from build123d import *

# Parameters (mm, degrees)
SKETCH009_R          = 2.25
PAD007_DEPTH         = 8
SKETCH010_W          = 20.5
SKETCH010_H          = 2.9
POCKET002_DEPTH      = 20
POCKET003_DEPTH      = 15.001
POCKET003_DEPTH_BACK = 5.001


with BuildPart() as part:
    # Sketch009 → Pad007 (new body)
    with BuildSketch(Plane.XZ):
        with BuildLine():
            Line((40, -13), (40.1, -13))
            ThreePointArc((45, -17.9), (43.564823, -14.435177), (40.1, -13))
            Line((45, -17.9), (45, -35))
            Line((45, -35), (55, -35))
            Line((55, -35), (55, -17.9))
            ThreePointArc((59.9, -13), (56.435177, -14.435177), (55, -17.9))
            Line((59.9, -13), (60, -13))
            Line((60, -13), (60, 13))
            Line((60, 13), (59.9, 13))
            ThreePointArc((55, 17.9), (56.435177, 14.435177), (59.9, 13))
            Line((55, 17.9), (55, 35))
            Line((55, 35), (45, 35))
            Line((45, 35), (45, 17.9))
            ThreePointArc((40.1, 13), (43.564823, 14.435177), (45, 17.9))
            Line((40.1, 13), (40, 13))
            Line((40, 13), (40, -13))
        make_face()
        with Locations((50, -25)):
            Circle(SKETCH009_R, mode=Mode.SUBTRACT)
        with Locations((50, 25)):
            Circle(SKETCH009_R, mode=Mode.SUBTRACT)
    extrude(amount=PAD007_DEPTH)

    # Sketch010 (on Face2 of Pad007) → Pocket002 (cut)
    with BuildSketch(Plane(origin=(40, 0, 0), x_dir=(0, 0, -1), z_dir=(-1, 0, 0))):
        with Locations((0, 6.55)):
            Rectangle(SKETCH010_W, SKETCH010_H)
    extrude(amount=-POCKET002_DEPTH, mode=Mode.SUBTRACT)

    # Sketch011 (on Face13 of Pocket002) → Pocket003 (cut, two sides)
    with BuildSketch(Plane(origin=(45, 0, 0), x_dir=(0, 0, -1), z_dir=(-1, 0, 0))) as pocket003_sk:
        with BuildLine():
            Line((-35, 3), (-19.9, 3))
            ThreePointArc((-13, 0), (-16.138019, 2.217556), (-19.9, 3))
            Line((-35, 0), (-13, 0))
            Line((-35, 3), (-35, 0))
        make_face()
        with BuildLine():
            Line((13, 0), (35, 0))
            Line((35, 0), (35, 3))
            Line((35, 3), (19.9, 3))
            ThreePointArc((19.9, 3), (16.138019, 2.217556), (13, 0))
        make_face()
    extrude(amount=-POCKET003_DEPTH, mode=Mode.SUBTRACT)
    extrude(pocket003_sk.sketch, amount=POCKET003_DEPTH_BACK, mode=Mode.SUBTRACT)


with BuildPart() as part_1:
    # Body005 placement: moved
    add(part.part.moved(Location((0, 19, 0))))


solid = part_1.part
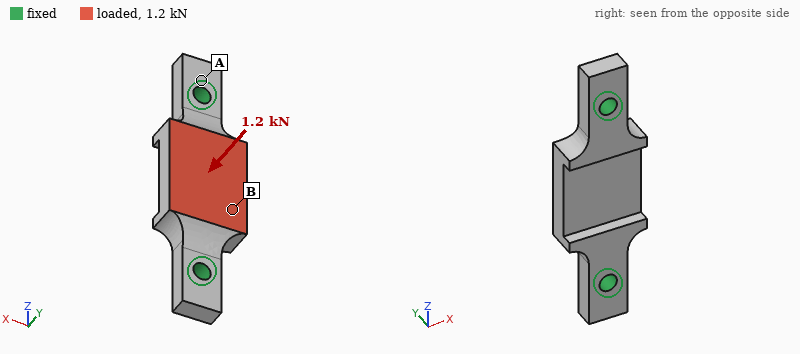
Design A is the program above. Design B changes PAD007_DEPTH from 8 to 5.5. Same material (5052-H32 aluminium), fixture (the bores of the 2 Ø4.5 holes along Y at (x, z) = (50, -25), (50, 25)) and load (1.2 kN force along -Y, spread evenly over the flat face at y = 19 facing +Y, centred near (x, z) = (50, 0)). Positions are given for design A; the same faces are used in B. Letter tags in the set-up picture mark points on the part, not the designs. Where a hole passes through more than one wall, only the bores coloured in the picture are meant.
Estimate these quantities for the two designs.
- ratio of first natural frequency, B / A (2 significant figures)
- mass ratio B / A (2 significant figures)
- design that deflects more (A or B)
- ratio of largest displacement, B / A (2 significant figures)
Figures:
0.57
0.75
B
2.5
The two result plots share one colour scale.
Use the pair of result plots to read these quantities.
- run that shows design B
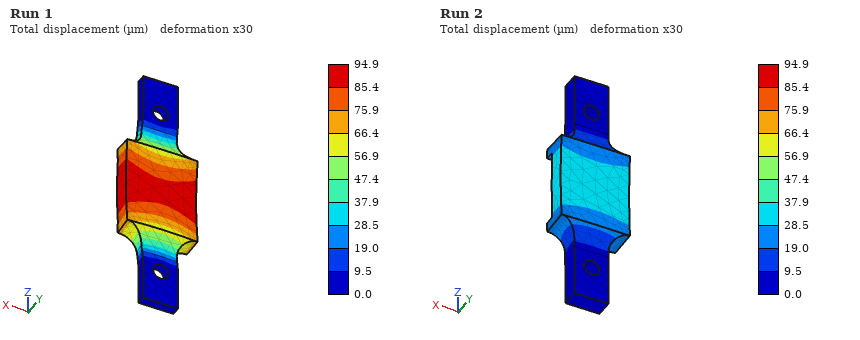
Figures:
Run 1
